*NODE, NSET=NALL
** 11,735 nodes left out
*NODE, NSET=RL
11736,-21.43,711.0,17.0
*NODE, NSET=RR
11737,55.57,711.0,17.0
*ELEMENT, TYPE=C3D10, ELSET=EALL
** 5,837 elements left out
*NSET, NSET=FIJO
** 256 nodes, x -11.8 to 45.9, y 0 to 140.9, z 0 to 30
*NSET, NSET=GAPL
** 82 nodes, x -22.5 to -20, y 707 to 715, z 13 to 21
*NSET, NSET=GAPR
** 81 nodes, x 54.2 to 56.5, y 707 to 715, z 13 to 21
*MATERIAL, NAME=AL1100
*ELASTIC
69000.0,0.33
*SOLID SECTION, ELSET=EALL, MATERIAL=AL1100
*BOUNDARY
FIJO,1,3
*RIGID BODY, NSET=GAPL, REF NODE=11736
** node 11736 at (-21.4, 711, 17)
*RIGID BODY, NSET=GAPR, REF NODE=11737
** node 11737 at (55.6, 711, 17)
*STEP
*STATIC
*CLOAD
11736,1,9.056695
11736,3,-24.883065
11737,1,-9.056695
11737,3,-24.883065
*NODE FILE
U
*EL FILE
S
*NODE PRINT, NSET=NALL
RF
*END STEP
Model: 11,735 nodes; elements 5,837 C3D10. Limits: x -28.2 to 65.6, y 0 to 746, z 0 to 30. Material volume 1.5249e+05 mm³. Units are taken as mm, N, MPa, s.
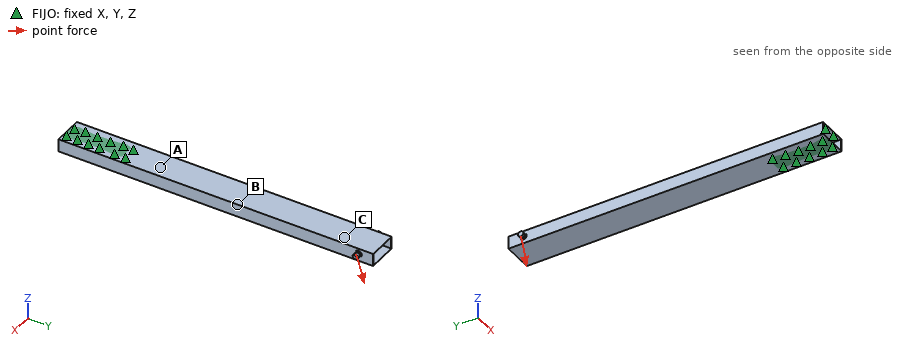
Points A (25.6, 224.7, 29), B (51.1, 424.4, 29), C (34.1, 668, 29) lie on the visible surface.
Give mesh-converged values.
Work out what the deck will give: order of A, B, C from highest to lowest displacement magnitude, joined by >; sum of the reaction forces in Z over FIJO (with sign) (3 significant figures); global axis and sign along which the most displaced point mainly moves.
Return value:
C > B > A
49.8 N
-Z
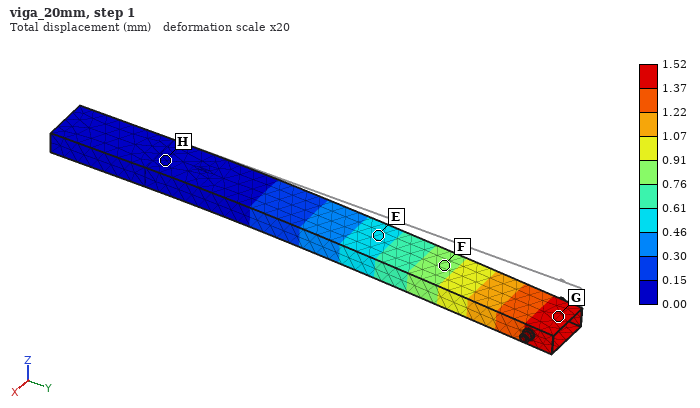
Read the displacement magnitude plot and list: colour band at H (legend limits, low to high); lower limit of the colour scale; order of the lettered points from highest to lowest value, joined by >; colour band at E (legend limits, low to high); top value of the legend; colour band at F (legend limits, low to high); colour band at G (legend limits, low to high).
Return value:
0.00 to 0.15 mm
0.00 mm
G > F > E > H
0.46 to 0.61 mm
1.52 mm
0.76 to 0.91 mm
1.37 to 1.52 mm
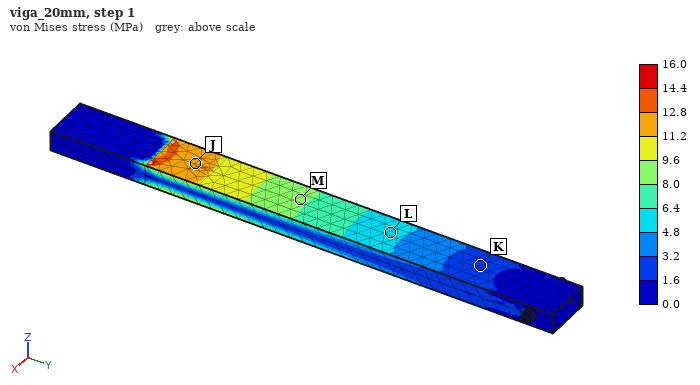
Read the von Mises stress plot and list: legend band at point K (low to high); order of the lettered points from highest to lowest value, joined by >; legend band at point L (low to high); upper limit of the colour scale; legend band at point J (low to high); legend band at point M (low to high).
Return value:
1.6 to 3.2 MPa
J > M > L > K
4.8 to 6.4 MPa
16.0 MPa
11.2 to 12.8 MPa
8.0 to 9.6 MPa
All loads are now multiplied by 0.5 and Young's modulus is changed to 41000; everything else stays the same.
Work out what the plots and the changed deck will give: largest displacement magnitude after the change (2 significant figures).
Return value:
1.3 mm
